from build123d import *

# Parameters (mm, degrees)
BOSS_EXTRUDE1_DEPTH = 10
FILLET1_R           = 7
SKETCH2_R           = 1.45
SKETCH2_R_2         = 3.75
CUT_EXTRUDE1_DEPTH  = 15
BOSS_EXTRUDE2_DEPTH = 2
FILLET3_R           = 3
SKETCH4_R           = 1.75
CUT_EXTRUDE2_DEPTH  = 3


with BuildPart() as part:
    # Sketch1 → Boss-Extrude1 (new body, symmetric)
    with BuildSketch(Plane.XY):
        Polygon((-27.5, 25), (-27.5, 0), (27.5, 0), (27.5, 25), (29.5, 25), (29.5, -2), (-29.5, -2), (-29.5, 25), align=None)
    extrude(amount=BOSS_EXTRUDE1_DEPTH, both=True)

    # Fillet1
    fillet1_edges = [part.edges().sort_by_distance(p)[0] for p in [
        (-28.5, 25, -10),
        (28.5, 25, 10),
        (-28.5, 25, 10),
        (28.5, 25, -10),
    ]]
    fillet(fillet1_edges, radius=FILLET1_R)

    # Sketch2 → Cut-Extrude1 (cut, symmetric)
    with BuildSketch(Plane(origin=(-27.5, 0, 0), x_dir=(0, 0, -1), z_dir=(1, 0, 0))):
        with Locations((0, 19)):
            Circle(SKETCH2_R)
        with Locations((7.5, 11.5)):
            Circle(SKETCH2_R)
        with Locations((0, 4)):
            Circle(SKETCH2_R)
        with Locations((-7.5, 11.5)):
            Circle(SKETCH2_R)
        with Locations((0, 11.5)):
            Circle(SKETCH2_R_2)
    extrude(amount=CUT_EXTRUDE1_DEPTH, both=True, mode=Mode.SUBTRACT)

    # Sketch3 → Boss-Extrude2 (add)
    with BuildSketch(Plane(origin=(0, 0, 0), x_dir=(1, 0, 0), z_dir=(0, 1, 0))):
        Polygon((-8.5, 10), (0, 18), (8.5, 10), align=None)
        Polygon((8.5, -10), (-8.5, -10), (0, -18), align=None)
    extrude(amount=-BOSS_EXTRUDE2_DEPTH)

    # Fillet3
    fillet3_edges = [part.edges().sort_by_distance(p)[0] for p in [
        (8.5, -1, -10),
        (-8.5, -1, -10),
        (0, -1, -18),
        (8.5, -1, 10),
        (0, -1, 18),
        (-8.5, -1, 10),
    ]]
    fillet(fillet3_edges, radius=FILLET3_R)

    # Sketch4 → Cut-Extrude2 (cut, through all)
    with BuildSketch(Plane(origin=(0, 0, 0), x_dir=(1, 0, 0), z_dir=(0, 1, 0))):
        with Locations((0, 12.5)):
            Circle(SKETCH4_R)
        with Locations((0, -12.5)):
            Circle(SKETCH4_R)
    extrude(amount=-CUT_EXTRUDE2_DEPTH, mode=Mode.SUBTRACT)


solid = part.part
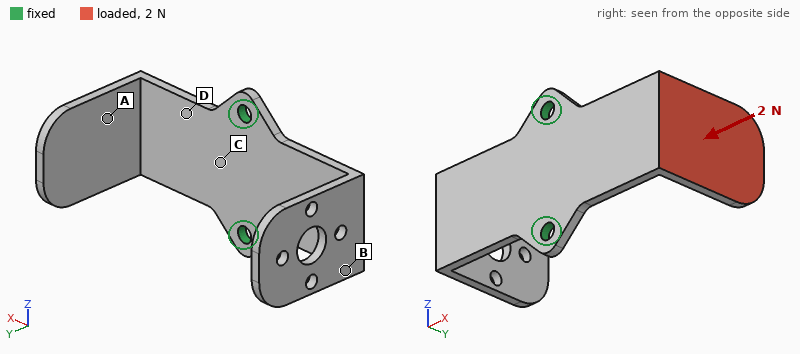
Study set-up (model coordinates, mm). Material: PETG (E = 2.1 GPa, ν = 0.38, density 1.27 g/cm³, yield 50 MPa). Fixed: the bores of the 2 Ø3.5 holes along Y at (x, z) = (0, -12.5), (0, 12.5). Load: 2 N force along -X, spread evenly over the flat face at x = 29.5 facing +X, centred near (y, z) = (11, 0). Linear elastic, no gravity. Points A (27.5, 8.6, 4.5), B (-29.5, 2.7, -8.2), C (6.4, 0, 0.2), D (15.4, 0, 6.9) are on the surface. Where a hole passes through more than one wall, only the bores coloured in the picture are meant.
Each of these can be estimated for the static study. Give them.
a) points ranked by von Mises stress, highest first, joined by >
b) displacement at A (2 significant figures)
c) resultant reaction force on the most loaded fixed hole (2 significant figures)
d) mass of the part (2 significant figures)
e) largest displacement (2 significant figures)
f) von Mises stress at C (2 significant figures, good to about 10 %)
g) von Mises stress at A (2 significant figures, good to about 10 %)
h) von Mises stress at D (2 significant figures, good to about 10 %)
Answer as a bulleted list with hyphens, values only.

- D > C > A > B
- 0.38 mm
- 1.0 N
- 5.5 g
- 0.79 mm
- 1.4 MPa
- 0.64 MPa
- 1.8 MPa
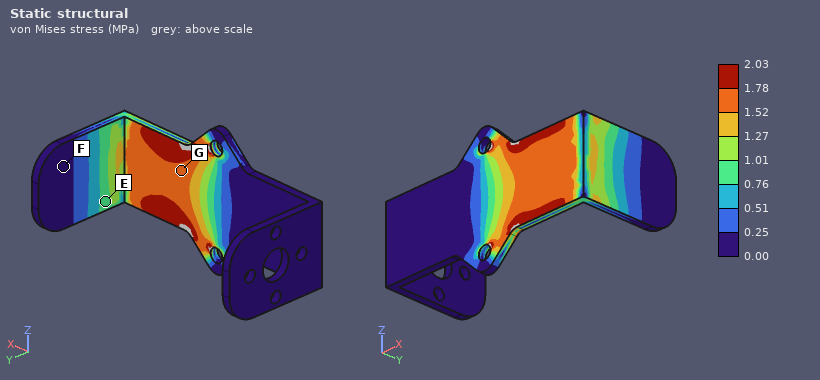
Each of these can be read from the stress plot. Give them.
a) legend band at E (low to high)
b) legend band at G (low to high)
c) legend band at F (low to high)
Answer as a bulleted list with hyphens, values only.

- 0.76 to 1.01 MPa
- 1.52 to 1.78 MPa
- 0.00 to 0.25 MPa
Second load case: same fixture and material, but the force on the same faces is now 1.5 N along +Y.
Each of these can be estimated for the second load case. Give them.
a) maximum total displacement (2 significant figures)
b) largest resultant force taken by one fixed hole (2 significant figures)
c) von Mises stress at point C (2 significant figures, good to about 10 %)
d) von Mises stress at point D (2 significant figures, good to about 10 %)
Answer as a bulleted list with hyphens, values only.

- 0.72 mm
- 0.75 N
- 1.9 MPa
- 1.6 MPa
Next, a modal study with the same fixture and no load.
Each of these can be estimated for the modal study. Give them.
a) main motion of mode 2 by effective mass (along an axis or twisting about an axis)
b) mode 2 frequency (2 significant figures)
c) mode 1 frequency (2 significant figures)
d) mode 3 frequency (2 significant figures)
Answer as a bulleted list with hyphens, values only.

- along Y
- 220 Hz
- 190 Hz
- 400 Hz
